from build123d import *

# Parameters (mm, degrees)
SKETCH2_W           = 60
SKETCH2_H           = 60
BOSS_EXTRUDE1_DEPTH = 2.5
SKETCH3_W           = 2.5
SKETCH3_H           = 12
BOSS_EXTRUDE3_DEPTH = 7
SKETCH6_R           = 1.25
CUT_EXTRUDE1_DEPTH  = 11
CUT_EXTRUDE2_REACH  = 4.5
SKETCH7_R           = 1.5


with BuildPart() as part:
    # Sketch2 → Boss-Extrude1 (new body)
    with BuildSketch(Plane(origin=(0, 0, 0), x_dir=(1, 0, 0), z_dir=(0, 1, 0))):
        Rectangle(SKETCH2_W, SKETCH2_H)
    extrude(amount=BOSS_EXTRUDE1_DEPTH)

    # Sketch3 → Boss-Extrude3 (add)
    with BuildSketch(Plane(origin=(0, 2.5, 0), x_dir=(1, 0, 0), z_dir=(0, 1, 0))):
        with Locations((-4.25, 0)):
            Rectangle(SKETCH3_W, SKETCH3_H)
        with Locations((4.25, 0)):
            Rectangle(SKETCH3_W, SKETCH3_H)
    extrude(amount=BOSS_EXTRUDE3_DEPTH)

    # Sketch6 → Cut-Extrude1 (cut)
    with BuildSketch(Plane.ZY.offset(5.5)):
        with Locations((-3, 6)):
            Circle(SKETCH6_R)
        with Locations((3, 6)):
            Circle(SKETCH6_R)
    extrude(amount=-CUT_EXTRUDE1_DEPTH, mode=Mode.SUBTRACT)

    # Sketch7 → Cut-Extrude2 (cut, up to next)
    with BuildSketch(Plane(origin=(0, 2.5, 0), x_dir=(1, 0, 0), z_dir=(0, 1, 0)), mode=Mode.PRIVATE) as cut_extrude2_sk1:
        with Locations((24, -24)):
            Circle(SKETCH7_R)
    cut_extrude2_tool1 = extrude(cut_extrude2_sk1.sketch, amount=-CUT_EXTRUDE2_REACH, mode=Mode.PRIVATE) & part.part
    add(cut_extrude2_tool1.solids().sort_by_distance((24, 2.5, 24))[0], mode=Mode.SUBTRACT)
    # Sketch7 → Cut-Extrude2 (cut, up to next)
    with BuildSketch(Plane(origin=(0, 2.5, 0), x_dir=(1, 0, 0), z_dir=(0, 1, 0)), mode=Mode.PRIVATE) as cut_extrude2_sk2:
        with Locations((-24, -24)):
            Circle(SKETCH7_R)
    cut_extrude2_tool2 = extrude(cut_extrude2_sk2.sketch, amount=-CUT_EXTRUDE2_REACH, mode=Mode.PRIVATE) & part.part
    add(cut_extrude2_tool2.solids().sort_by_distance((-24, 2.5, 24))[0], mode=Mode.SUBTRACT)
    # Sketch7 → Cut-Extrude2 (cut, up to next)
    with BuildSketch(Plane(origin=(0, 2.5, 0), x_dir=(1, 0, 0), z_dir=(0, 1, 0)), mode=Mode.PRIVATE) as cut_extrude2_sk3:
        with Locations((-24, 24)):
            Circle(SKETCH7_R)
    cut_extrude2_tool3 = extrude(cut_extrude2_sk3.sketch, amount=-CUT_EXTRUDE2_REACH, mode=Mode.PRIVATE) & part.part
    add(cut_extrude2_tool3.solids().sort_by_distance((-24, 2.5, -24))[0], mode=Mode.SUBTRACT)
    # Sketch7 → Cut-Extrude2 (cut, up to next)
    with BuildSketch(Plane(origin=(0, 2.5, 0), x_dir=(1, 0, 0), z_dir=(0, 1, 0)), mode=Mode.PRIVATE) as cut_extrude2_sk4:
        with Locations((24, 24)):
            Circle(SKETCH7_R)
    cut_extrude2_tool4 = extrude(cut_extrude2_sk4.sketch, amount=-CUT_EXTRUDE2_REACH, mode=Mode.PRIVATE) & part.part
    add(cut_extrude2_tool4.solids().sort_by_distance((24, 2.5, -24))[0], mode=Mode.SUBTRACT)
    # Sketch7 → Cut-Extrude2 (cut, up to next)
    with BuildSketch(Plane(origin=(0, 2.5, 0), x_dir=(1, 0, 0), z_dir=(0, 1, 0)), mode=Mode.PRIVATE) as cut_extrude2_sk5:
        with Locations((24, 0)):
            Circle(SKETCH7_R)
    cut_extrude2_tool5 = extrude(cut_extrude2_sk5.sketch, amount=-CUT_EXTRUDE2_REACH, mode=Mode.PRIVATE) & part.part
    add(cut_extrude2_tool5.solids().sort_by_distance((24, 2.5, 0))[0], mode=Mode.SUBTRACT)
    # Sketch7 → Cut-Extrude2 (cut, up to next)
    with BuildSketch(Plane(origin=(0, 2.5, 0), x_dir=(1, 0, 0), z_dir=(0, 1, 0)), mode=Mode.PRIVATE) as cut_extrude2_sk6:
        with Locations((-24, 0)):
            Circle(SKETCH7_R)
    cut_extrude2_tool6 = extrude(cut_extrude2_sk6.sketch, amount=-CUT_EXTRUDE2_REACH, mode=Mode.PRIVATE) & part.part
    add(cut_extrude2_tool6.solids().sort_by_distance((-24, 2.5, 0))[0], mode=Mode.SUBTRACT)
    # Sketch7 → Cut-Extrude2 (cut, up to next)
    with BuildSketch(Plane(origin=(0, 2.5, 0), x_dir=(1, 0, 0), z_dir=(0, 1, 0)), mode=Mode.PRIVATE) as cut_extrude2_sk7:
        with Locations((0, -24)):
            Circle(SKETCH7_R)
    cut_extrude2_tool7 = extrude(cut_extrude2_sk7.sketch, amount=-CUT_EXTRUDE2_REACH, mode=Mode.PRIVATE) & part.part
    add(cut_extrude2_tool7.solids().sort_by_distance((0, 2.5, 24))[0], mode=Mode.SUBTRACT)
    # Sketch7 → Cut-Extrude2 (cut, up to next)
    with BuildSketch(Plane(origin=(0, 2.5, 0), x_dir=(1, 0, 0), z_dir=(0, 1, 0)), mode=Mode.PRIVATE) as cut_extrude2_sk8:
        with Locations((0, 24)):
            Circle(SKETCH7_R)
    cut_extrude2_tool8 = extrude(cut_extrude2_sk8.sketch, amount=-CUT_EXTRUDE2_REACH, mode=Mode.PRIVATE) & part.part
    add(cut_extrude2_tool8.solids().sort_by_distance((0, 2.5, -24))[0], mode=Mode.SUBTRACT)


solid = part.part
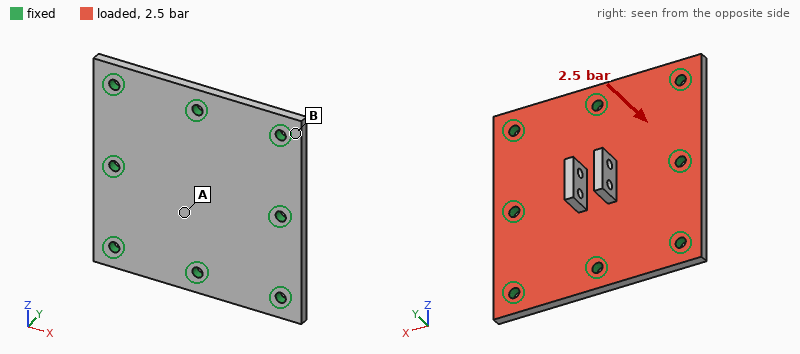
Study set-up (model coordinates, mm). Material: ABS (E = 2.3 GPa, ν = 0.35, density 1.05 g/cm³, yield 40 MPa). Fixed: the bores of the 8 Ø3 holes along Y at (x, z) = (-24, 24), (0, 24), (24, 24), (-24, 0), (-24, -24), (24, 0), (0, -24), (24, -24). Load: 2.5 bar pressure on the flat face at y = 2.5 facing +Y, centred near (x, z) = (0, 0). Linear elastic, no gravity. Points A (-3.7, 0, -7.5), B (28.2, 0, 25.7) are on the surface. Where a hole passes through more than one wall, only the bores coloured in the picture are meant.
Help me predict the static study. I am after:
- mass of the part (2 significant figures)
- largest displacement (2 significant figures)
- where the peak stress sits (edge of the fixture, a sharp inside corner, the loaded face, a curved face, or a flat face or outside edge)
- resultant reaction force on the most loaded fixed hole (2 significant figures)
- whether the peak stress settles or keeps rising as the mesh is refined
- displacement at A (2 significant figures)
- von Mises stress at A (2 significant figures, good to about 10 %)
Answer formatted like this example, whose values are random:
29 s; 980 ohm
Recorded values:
9.7 g; 0.51 mm; edge of the fixture; 150 N; keeps rising; 0.45 mm; 12 MPa
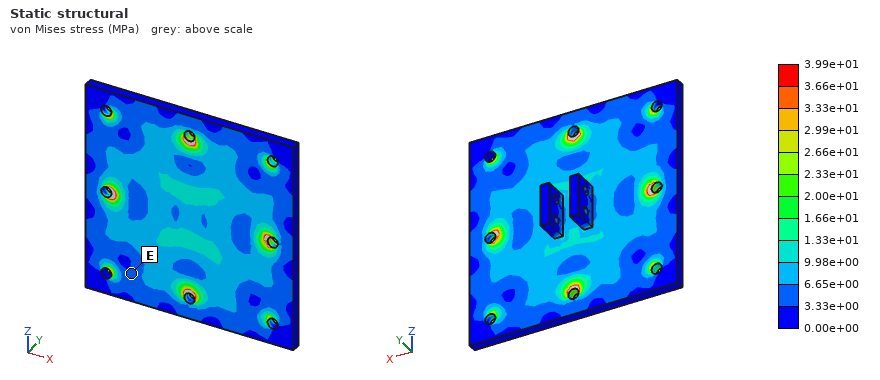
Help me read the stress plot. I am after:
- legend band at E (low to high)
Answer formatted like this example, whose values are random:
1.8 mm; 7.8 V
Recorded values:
3.33e+00 to 6.65e+00 MPa
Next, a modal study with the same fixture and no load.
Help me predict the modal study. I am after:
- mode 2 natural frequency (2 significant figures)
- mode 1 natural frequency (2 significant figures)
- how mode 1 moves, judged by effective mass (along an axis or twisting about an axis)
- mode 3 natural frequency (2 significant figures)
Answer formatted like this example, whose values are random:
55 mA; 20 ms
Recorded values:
4200 Hz; 2300 Hz; along Y; 4200 Hz
